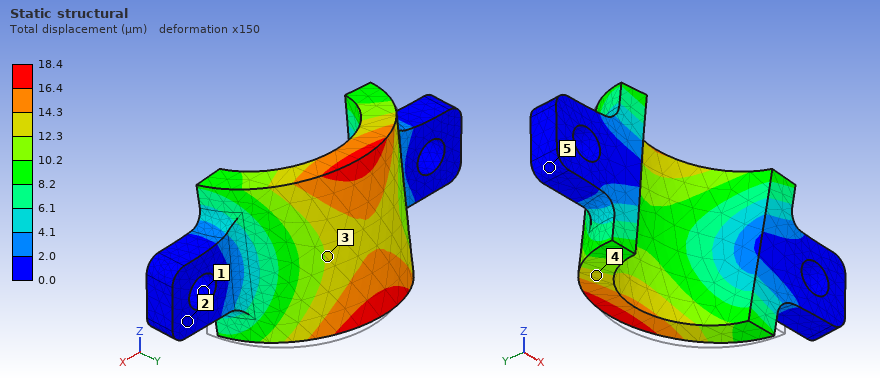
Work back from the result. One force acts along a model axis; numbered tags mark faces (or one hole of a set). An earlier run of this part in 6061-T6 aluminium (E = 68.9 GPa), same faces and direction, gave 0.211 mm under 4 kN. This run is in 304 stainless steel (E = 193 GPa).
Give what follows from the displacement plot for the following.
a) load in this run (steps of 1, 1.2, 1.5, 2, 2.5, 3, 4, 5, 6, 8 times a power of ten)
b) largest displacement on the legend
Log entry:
1 kN
18.4 µm
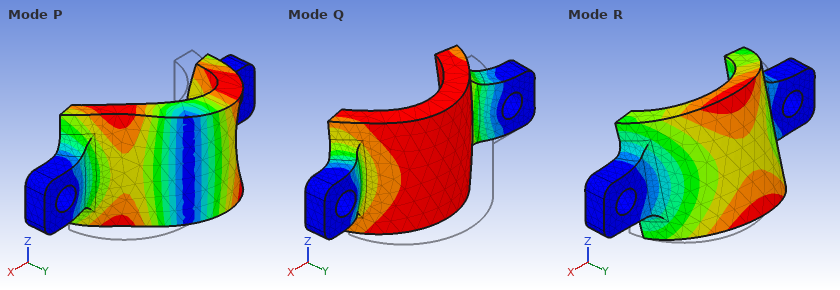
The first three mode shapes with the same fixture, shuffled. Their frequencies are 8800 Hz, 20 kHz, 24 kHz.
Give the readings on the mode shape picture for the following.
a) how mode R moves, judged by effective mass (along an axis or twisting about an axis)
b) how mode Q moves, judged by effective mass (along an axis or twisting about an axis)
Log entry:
along Z
along Y
